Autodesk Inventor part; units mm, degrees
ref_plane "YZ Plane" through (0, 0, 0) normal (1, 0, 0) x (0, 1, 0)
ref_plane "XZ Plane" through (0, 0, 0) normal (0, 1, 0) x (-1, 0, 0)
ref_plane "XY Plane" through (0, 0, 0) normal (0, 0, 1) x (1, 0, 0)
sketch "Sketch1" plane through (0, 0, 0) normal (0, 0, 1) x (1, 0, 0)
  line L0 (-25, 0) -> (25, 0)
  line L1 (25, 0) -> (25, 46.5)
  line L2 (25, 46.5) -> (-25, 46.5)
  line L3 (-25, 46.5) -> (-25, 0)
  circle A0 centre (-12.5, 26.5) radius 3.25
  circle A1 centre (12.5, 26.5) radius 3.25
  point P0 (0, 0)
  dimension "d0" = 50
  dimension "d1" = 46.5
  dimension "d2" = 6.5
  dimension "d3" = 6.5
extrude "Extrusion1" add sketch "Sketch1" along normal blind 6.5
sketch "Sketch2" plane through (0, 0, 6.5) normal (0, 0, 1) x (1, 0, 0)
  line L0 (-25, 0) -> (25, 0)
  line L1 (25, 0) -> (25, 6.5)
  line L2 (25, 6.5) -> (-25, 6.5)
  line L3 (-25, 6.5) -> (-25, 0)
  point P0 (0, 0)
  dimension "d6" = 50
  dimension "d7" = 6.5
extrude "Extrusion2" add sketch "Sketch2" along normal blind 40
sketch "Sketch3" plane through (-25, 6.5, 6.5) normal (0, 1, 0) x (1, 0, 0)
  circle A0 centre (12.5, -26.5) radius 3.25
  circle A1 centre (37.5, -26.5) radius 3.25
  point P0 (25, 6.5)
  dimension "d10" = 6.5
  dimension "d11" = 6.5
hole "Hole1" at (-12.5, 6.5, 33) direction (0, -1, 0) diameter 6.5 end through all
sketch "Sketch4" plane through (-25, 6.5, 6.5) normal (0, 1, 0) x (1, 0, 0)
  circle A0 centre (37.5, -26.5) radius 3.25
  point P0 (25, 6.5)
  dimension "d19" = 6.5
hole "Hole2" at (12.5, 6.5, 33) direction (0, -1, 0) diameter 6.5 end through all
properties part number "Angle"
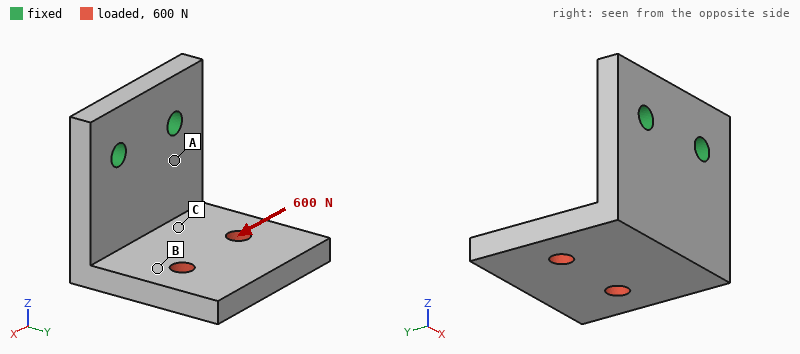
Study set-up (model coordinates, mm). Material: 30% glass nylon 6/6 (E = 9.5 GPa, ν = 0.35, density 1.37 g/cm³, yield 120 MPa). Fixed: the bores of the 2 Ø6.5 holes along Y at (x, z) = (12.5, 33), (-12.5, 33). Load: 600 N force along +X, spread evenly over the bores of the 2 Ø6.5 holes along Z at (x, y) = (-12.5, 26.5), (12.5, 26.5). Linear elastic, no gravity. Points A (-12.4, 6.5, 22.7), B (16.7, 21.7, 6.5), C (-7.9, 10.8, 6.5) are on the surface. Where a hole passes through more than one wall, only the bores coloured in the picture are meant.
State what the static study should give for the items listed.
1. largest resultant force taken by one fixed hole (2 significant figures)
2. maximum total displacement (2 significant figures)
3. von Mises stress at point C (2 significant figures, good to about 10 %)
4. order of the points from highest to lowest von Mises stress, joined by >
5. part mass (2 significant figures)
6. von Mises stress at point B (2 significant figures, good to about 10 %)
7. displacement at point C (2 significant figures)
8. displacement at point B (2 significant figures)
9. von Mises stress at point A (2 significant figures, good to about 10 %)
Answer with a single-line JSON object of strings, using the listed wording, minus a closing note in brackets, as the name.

{"largest resultant force taken by one fixed hole": "780 N", "maximum total displacement": "0.69 mm", "von Mises stress at point C": "14 MPa", "order of the points from highest to lowest von Mises stress, joined by >": "A > C > B", "part mass": "37 g", "von Mises stress at point B": "6.2 MPa", "displacement at point C": "0.16 mm", "displacement at point B": "0.35 mm", "von Mises stress at point A": "22 MPa"}
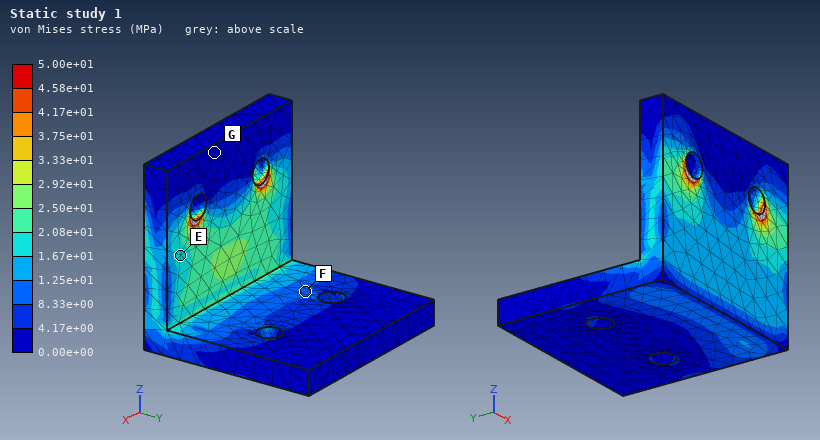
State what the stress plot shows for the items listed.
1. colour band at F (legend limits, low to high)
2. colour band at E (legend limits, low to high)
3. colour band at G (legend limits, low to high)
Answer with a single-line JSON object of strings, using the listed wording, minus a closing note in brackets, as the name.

{"colour band at F": "8.33e+00 to 1.25e+01 MPa", "colour band at E": "1.67e+01 to 2.08e+01 MPa", "colour band at G": "0.00e+00 to 4.17e+00 MPa"}
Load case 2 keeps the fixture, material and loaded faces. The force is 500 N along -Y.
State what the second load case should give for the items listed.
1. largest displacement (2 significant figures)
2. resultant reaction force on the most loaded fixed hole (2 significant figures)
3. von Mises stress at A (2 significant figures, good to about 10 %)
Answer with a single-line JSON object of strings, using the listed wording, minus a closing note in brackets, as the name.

{"largest displacement": "0.91 mm", "resultant reaction force on the most loaded fixed hole": "250 N", "von Mises stress at A": "27 MPa"}
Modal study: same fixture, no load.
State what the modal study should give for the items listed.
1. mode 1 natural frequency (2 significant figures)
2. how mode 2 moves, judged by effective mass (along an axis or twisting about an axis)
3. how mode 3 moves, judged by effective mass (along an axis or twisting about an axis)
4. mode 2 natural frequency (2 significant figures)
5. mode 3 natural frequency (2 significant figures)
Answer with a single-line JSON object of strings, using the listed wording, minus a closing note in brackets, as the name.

{"mode 1 natural frequency": "720 Hz", "how mode 2 moves, judged by effective mass": "along X", "how mode 3 moves, judged by effective mass": "along Y", "mode 2 natural frequency": "1200 Hz", "mode 3 natural frequency": "2100 Hz"}
